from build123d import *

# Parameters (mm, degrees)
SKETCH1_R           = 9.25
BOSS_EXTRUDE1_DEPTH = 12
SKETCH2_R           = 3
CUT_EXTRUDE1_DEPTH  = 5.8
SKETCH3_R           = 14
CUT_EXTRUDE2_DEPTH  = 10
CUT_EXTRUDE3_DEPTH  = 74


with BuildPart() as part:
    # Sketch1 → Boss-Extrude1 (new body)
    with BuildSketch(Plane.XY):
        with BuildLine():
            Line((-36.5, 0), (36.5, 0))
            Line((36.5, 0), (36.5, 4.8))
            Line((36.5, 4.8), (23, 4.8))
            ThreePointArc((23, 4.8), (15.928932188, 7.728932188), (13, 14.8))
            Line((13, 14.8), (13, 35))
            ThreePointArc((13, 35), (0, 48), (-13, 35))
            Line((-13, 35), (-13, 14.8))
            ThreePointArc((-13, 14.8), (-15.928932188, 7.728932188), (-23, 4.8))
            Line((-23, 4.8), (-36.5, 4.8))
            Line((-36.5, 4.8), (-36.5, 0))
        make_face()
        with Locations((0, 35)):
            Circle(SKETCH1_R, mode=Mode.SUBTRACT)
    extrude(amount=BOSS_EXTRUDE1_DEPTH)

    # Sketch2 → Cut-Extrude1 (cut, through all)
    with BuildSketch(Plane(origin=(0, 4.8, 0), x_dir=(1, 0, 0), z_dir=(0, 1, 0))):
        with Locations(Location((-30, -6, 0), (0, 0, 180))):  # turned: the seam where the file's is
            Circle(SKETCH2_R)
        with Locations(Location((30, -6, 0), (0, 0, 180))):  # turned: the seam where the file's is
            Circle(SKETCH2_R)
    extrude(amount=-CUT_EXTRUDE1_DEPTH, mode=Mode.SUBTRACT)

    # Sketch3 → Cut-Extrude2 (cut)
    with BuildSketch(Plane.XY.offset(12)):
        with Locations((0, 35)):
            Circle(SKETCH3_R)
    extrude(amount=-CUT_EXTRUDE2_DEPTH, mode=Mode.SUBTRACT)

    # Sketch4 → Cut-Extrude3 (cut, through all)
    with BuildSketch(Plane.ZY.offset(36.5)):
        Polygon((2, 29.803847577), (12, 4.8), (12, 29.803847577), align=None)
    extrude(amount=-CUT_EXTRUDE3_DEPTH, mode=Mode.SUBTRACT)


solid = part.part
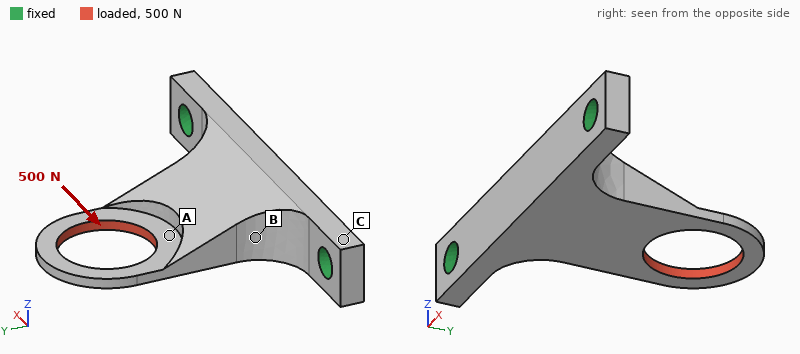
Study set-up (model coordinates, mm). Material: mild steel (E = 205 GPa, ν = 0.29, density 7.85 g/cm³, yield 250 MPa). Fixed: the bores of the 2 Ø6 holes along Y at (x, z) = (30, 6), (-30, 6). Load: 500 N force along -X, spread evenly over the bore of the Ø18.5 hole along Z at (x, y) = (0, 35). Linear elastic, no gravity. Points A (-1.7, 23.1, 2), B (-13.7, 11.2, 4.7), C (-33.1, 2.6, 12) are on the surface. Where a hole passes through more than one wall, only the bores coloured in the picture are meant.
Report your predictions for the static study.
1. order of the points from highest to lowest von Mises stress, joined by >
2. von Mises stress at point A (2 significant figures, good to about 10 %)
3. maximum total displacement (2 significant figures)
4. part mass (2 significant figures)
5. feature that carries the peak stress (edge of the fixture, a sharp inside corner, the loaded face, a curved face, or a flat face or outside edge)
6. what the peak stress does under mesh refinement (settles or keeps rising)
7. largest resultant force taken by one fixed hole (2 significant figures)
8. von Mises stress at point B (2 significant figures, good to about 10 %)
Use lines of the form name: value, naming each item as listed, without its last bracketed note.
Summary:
order of the points from highest to lowest von Mises stress, joined by >: A > B > C
von Mises stress at point A: 42 MPa
maximum total displacement: 37 µm
part mass: 71 g
feature that carries the peak stress: a sharp inside corner
what the peak stress does under mesh refinement: keeps rising
largest resultant force taken by one fixed hole: 440 N
von Mises stress at point B: 23 MPa
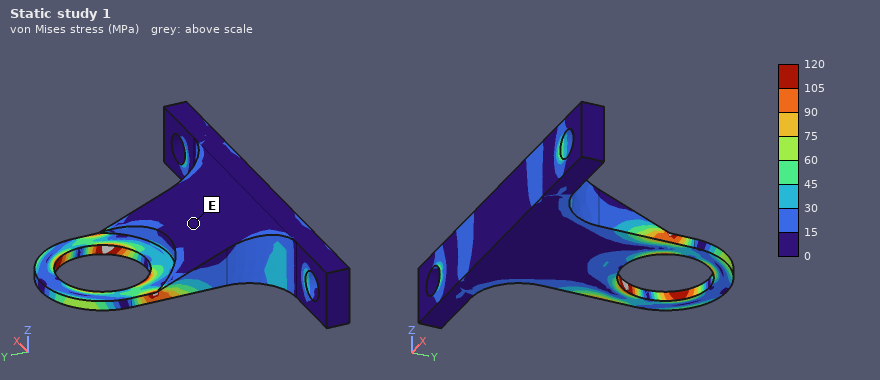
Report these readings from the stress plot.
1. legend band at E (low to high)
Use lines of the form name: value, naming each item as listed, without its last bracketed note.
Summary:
legend band at E: 0 to 15 MPa
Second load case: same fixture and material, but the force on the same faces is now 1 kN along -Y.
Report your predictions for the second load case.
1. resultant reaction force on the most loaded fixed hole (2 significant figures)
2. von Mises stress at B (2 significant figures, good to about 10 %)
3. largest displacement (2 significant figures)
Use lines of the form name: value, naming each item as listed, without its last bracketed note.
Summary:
resultant reaction force on the most loaded fixed hole: 660 N
von Mises stress at B: 26 MPa
largest displacement: 62 µm
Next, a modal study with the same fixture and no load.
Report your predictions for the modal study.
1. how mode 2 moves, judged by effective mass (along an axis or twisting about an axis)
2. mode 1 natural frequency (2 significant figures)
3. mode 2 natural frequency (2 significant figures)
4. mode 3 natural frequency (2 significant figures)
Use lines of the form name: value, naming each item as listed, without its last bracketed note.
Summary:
how mode 2 moves, judged by effective mass: along Z
mode 1 natural frequency: 2500 Hz
mode 2 natural frequency: 5000 Hz
mode 3 natural frequency: 7400 Hz
